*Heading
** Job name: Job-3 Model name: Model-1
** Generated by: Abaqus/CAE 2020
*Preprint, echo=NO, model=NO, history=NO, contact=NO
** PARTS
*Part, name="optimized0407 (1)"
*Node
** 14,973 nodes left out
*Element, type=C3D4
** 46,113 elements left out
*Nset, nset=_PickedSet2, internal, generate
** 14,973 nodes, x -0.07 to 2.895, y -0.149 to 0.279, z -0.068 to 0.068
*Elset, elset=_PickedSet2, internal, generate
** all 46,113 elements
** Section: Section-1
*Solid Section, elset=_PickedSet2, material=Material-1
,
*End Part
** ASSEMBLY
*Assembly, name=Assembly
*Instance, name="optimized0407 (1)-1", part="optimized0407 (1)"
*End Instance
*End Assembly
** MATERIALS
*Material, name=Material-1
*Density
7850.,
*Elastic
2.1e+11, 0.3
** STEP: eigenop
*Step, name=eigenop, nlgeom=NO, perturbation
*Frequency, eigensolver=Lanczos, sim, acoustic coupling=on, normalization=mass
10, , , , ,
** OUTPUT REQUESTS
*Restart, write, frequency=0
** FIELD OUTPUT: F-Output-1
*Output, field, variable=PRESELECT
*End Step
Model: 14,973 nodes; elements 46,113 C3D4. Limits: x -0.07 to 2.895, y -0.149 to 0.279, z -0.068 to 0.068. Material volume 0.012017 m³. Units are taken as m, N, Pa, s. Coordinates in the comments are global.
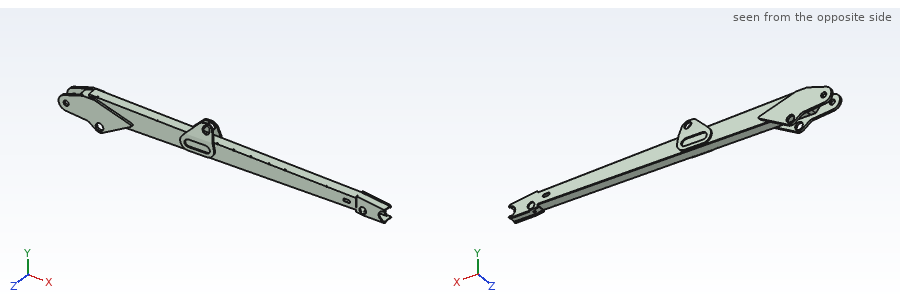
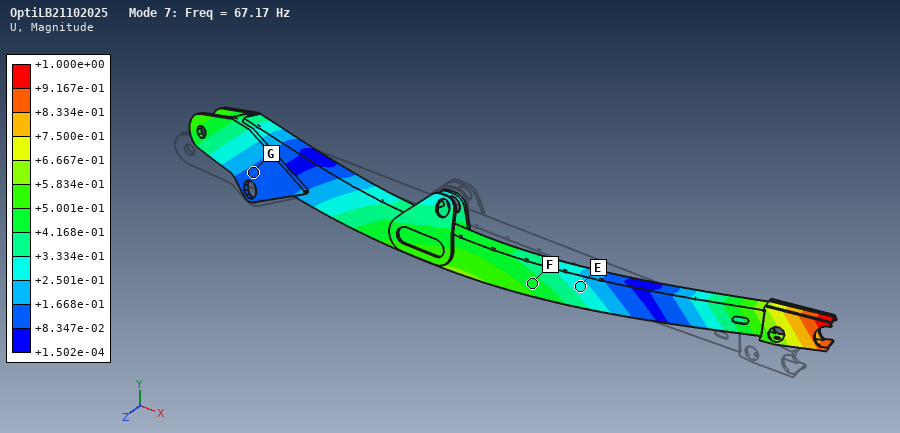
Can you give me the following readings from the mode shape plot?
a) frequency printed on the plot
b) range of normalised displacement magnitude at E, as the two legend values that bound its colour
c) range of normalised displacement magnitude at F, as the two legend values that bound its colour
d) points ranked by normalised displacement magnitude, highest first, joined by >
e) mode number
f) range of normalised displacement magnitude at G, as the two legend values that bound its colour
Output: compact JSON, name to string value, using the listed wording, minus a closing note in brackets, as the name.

{"frequency printed on the plot": "67.17 Hz", "range of normalised displacement magnitude at E, as the two legend values that bound its colour": "+2.501e-01 to +3.334e-01", "range of normalised displacement magnitude at F, as the two legend values that bound its colour": "+4.168e-01 to +5.001e-01", "points ranked by normalised displacement magnitude, highest first, joined by >": "F > E > G", "mode number": "7", "range of normalised displacement magnitude at G, as the two legend values that bound its colour": "+8.347e-02 to +1.668e-01"}
